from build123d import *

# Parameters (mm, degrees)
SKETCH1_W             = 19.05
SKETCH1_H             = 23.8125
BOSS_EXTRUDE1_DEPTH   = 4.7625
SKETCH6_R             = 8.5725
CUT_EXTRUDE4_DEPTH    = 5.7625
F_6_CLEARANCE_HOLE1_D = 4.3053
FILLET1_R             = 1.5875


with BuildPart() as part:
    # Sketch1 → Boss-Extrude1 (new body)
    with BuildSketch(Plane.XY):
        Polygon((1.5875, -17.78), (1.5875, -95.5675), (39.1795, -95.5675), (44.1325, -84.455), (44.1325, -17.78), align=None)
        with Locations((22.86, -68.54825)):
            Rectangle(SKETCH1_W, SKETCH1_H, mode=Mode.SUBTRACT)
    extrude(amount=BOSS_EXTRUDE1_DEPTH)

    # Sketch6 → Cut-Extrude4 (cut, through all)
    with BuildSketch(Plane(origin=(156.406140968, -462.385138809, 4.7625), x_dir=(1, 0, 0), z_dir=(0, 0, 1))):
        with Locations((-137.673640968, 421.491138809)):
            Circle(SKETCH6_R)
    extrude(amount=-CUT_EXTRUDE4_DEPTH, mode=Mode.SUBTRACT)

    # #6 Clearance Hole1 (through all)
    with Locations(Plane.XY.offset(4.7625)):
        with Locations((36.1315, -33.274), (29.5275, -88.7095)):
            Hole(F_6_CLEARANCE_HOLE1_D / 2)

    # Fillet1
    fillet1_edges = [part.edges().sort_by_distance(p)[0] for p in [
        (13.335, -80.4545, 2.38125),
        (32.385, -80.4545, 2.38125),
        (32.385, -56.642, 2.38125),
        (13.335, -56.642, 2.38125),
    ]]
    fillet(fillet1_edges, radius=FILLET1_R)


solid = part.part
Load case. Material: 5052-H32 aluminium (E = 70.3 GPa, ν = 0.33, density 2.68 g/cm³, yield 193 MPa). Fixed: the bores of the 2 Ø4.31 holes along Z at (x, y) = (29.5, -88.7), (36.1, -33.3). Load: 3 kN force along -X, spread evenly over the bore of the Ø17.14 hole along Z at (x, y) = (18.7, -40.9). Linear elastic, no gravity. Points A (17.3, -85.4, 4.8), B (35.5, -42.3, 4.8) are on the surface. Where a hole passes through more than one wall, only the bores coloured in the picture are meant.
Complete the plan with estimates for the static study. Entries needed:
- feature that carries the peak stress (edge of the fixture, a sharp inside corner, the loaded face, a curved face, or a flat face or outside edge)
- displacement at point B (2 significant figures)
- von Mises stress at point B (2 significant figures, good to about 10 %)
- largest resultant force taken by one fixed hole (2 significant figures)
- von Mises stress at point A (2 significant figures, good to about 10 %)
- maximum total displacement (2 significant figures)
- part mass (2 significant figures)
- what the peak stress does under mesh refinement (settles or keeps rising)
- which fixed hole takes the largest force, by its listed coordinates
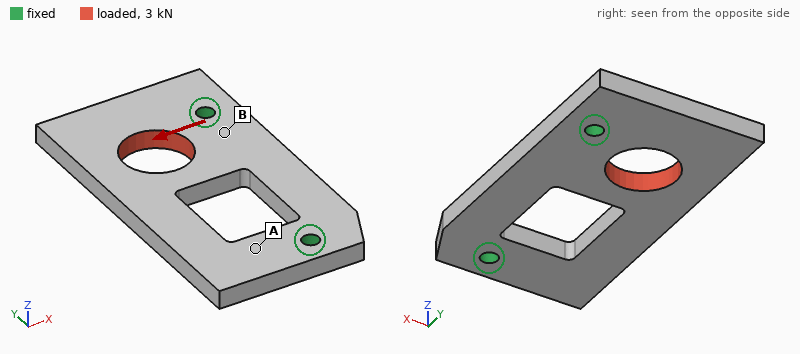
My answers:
edge of the fixture
8.0 µm
24 MPa
2.6 kN
10 MPa
24 µm
33 g
keeps rising
(36.1, -33.3)
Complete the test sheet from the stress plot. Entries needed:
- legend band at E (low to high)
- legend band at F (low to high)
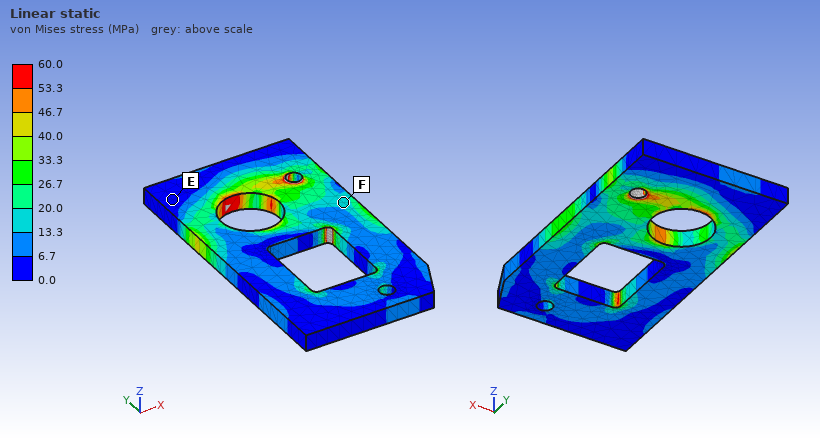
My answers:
0.0 to 6.7 MPa
13.3 to 20.0 MPa
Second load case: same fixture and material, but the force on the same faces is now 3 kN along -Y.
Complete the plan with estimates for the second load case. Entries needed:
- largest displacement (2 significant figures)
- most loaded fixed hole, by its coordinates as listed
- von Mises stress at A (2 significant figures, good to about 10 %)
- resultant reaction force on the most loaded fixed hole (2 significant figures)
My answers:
44 µm
(36.1, -33.3)
32 MPa
2.1 kN
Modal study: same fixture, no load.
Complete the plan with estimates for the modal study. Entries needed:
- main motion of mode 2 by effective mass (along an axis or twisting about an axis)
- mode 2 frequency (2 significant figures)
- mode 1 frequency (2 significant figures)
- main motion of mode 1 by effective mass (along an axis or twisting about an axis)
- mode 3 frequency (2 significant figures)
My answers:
twisting about X
4500 Hz
2700 Hz
along Z
6800 Hz
